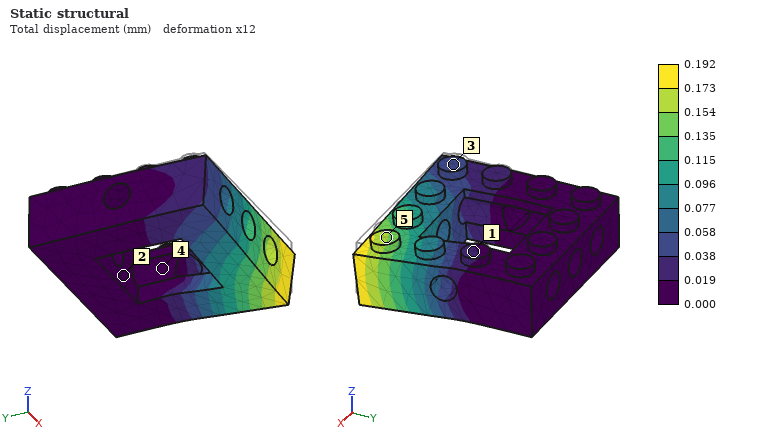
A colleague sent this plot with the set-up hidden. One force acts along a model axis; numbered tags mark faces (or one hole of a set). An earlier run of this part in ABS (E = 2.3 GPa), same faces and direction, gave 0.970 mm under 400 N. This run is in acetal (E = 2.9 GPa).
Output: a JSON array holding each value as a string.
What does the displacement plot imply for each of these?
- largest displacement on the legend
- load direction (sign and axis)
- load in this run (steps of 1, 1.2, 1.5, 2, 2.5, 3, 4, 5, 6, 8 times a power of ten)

["0.192 mm", "-Z", "100 N"]
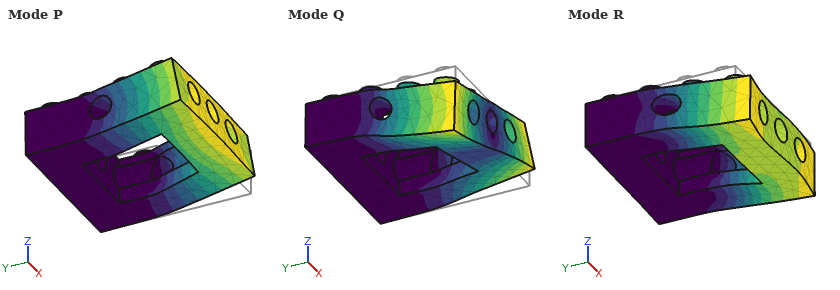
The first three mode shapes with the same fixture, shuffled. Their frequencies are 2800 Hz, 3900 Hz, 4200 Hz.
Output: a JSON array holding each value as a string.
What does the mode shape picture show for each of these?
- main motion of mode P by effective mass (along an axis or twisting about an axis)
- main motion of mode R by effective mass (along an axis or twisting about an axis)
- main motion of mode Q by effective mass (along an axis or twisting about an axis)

["along Z", "along X", "twisting about Y"]
